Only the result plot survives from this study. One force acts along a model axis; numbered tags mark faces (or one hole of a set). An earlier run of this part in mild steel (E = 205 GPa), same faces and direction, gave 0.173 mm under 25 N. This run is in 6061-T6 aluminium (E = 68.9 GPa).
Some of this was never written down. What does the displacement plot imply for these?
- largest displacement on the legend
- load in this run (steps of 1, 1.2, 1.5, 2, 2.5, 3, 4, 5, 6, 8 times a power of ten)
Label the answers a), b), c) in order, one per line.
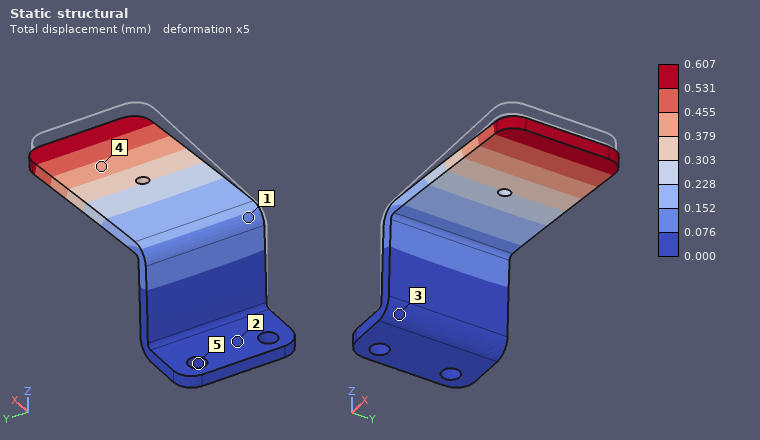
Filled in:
a) 0.607 mm
b) 30 N
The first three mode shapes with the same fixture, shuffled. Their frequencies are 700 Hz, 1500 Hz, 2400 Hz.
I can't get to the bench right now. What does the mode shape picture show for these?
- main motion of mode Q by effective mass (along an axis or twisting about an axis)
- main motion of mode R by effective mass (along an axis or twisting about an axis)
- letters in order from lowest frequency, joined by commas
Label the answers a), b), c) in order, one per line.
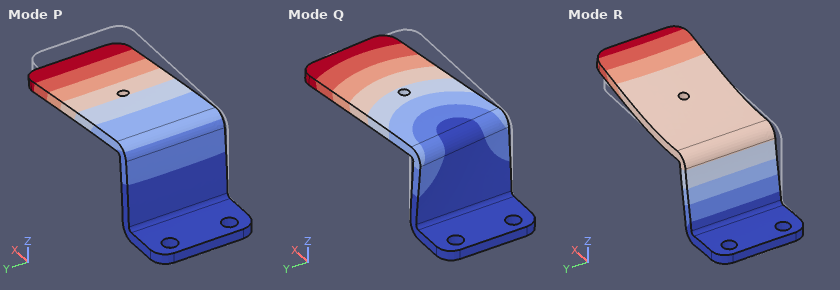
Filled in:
a) along Y
b) along X
c) P, Q, R
